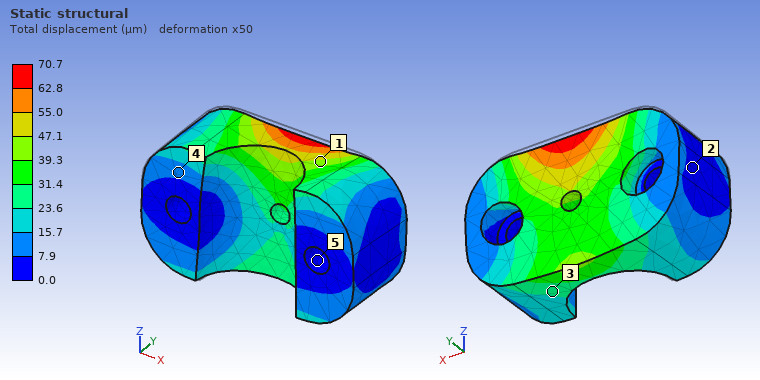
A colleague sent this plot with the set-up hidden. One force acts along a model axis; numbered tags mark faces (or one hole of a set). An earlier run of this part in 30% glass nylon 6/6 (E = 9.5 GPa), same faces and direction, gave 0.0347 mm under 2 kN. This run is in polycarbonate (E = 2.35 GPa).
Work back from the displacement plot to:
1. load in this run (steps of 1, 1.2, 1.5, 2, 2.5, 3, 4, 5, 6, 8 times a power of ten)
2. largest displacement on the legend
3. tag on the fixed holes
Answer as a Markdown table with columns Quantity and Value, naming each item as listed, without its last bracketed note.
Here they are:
| Quantity | Value |
|---|---|
| load in this run | 1 kN |
| largest displacement on the legend | 70.7 µm |
| tag on the fixed holes | 5 |
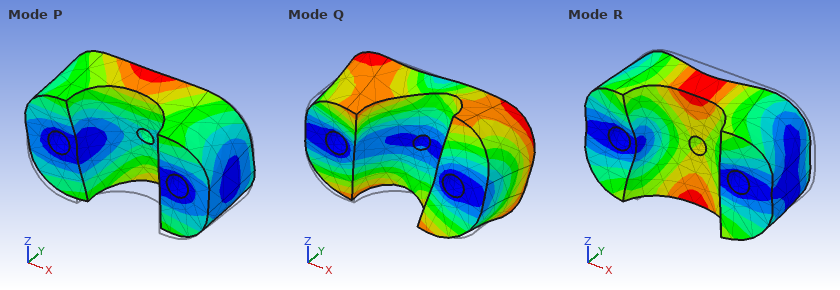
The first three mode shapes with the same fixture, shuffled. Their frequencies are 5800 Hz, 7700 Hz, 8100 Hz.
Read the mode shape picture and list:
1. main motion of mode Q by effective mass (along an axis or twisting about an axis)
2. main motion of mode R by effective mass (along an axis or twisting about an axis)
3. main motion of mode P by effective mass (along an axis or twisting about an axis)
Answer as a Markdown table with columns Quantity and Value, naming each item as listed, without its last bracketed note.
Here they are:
| Quantity | Value |
|---|---|
| main motion of mode Q by effective mass | twisting about Y |
| main motion of mode R by effective mass | along Y |
| main motion of mode P by effective mass | along Z |
